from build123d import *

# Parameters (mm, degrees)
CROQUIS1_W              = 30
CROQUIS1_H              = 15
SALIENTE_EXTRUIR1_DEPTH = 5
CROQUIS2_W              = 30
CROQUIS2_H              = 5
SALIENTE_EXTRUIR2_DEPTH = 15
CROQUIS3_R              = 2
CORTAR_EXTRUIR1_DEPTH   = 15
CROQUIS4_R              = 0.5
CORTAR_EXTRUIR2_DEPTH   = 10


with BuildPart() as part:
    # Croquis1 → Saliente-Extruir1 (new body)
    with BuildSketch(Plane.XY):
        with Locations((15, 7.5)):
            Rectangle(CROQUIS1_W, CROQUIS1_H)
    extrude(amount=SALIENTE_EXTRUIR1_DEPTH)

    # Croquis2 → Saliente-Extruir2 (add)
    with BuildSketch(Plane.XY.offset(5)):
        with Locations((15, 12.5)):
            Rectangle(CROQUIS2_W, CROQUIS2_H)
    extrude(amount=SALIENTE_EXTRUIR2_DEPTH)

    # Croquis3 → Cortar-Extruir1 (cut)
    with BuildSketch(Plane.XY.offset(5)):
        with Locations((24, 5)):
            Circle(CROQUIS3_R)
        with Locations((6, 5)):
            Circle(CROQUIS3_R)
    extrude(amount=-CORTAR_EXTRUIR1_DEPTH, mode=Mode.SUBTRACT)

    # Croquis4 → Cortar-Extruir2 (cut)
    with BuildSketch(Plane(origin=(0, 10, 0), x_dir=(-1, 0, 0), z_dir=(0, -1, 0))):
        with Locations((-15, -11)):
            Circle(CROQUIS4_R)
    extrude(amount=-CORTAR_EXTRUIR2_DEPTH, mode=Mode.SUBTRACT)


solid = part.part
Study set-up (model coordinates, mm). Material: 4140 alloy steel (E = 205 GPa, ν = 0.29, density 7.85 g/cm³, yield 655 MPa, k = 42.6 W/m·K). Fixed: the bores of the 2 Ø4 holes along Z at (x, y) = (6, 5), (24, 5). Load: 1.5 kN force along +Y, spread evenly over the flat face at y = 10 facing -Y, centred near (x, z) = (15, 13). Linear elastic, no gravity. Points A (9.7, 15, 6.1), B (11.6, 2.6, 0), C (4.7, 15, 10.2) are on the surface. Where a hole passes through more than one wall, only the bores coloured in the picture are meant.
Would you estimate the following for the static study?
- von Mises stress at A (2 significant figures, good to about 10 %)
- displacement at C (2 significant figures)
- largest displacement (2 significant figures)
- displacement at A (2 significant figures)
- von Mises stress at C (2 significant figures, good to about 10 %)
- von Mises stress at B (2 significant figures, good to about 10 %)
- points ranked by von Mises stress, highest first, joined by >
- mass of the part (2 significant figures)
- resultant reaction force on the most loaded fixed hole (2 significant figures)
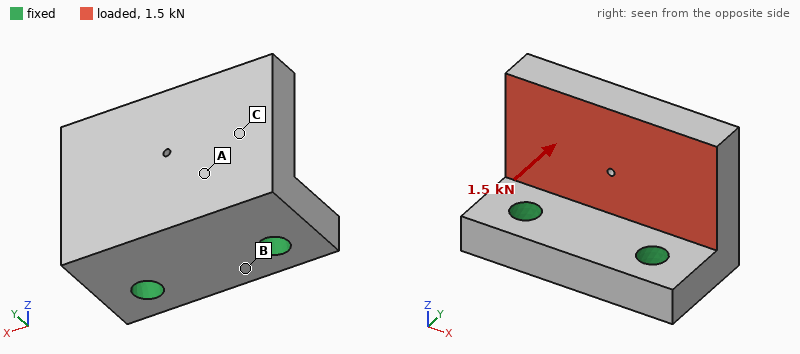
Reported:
70 MPa
20 µm
43 µm
13 µm
38 MPa
18 MPa
A > C > B
34 g
760 N
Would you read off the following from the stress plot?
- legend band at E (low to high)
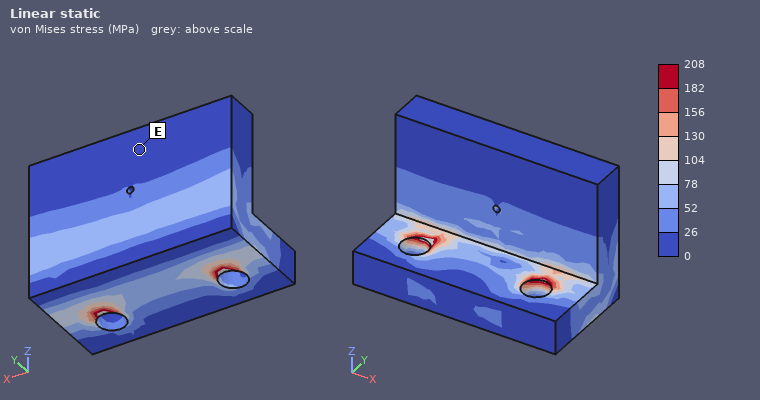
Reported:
0 to 26 MPa
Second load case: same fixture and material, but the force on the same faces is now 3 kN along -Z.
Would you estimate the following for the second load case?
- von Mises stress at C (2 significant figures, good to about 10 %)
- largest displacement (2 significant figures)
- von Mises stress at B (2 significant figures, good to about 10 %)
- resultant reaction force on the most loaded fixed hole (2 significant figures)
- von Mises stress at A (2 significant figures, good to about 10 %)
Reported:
24 MPa
6.9 µm
20 MPa
1.5 kN
29 MPa
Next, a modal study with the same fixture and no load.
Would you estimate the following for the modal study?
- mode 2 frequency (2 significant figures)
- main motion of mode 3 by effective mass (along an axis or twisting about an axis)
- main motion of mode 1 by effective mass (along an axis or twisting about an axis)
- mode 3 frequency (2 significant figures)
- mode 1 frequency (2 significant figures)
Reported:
15 kHz
along X
along Y
21 kHz
8400 Hz
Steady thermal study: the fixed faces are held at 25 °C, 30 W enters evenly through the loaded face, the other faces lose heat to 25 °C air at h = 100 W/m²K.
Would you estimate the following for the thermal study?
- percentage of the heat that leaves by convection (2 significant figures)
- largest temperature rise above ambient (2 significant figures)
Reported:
18 %
63 K
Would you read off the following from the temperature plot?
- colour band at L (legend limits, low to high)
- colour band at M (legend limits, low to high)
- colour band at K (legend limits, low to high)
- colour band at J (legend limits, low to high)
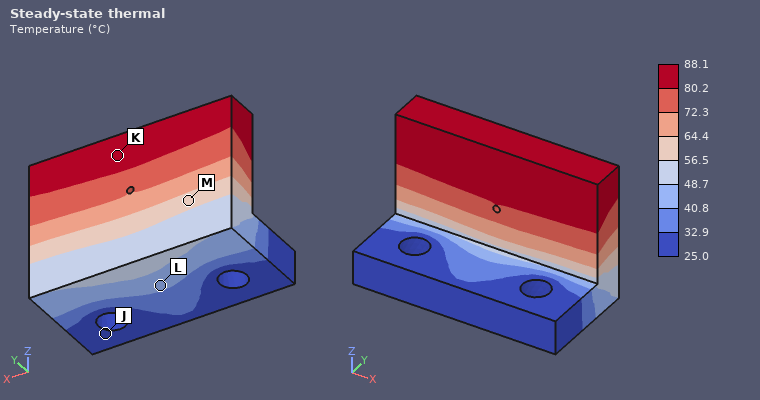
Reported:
40.8 to 48.7 °C
56.5 to 64.4 °C
80.2 to 88.1 °C
25.0 to 32.9 °C
